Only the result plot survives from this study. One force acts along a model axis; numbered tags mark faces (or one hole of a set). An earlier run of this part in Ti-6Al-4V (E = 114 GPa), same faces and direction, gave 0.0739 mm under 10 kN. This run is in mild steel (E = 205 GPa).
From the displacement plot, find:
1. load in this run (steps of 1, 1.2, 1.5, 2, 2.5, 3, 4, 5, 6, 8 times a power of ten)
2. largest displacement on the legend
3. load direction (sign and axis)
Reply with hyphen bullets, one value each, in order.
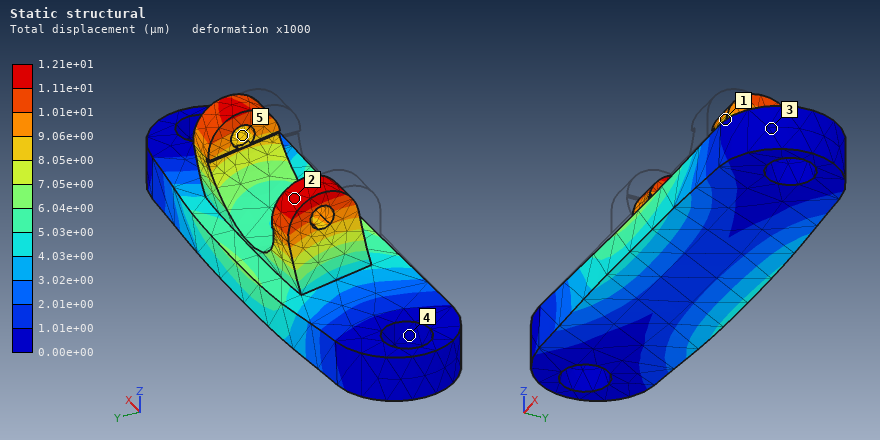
- 3 kN
- 1.21e+01 µm
- +Y
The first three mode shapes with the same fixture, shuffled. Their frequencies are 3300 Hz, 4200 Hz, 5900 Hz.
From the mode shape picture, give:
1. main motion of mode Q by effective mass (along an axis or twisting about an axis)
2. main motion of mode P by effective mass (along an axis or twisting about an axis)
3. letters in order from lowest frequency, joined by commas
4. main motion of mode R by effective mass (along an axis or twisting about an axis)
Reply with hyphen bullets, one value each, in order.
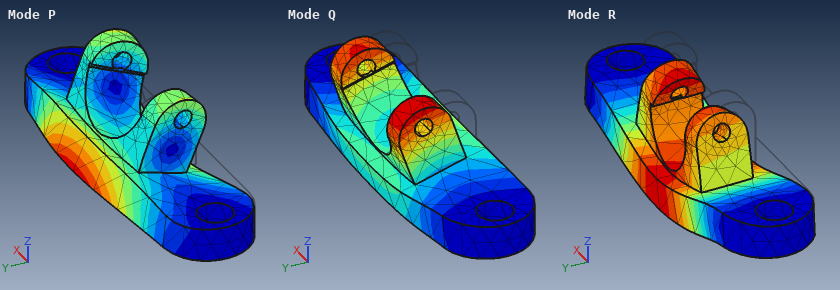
- along Y
- along Y
- R, Q, P
- along Z
